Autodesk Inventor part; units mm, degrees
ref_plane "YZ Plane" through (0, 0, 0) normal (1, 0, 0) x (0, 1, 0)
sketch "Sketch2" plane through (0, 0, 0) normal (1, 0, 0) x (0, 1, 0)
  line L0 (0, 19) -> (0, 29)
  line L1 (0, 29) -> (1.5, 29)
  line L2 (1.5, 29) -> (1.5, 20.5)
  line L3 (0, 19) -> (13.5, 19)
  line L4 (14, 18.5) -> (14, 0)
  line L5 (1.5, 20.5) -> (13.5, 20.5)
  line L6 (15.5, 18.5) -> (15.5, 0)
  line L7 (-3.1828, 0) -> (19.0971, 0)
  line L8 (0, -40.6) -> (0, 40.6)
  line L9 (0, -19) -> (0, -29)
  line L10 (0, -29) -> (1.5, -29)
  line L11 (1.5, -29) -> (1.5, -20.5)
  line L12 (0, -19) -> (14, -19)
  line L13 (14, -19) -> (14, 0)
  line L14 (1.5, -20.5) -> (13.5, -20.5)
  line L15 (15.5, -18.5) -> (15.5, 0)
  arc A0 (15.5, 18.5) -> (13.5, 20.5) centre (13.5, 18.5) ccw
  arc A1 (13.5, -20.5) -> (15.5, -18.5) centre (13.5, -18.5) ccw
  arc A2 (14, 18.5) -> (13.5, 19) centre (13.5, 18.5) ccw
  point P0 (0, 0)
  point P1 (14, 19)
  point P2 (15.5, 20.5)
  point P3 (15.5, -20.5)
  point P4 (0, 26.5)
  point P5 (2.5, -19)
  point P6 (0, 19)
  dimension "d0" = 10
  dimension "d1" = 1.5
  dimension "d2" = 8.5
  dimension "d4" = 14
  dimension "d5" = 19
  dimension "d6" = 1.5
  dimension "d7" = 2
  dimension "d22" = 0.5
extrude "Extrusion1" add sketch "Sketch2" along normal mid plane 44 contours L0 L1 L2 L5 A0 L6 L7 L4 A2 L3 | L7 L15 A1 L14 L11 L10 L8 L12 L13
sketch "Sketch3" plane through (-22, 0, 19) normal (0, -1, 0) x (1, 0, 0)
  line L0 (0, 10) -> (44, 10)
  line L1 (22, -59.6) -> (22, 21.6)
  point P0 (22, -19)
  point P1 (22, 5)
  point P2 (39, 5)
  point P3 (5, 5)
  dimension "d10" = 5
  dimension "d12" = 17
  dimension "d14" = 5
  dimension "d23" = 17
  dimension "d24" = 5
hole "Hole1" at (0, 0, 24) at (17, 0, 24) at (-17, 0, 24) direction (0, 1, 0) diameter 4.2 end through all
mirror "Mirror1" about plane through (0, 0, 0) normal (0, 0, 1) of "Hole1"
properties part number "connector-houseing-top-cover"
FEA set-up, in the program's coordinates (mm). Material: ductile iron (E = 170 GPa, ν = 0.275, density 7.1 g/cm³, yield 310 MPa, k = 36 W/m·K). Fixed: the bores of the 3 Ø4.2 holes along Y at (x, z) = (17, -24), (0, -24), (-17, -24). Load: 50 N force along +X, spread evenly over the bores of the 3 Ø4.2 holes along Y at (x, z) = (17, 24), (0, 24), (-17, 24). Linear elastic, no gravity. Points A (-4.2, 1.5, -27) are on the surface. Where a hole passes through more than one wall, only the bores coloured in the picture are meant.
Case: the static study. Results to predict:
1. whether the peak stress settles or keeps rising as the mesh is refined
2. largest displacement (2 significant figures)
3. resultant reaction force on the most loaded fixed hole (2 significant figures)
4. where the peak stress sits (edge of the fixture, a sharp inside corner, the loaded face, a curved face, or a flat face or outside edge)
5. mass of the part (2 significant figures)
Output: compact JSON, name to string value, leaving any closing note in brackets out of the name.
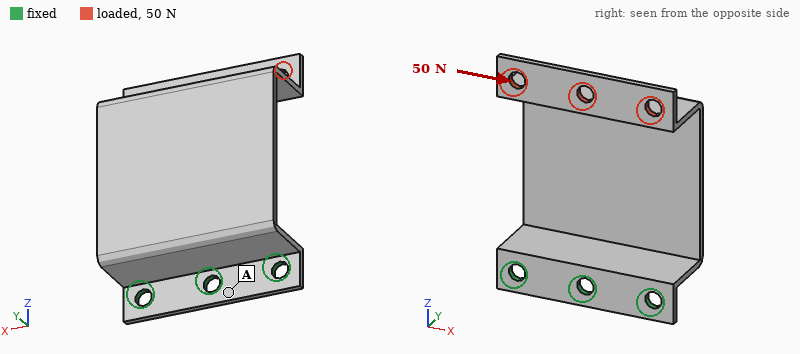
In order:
{"whether the peak stress settles or keeps rising as the mesh is refined": "keeps rising", "largest displacement": "0.36 mm", "resultant reaction force on the most loaded fixed hole": "67 N", "where the peak stress sits": "edge of the fixture", "mass of the part": "39 g"}
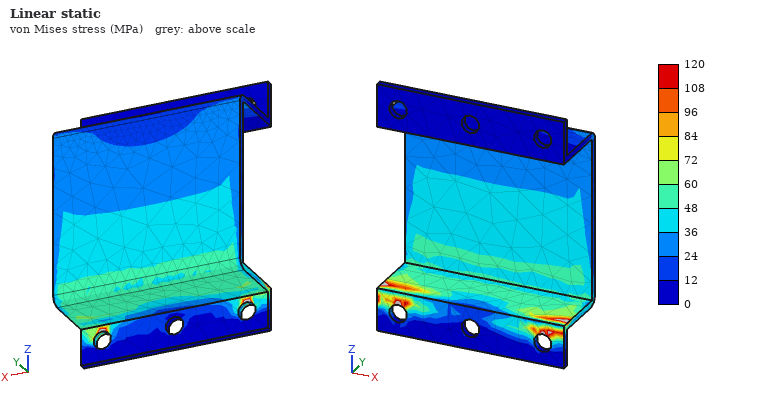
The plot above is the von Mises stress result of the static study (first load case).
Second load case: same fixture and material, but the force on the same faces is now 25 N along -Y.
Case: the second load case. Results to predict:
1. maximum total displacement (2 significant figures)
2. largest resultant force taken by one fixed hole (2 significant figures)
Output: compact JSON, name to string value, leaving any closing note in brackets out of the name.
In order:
{"maximum total displacement": "0.79 mm", "largest resultant force taken by one fixed hole": "14 N"}
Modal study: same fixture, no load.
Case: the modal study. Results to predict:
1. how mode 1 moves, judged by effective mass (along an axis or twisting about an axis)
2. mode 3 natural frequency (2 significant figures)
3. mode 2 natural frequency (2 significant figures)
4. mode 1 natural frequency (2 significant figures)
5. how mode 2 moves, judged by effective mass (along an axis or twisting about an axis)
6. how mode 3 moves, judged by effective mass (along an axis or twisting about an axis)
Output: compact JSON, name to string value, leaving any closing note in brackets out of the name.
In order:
{"how mode 1 moves, judged by effective mass": "along Y", "mode 3 natural frequency": "1100 Hz", "mode 2 natural frequency": "600 Hz", "mode 1 natural frequency": "260 Hz", "how mode 2 moves, judged by effective mass": "along X", "how mode 3 moves, judged by effective mass": "along Z"}
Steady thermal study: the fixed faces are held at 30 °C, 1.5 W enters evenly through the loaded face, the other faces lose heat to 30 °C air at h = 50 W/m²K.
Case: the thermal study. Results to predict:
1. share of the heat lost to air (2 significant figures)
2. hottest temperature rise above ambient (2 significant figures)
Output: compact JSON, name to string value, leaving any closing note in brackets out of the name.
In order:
{"share of the heat lost to air": "94 %", "hottest temperature rise above ambient": "14 K"}
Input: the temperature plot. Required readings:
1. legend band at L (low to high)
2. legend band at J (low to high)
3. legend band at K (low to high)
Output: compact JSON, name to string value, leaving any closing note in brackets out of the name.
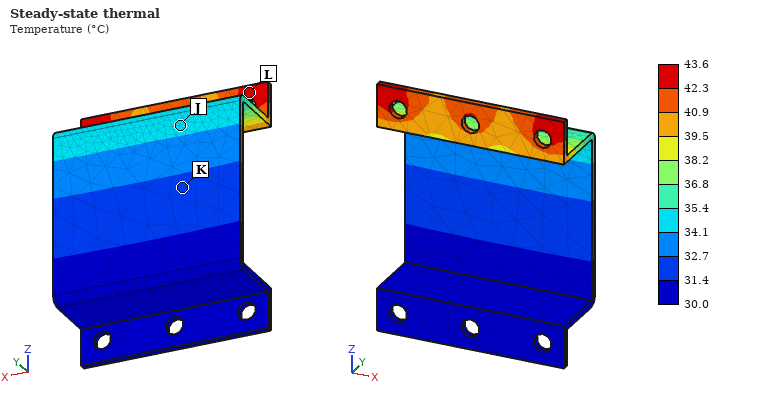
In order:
{"legend band at L": "42.3 to 43.6 °C", "legend band at J": "34.1 to 35.4 °C", "legend band at K": "31.4 to 32.7 °C"}
